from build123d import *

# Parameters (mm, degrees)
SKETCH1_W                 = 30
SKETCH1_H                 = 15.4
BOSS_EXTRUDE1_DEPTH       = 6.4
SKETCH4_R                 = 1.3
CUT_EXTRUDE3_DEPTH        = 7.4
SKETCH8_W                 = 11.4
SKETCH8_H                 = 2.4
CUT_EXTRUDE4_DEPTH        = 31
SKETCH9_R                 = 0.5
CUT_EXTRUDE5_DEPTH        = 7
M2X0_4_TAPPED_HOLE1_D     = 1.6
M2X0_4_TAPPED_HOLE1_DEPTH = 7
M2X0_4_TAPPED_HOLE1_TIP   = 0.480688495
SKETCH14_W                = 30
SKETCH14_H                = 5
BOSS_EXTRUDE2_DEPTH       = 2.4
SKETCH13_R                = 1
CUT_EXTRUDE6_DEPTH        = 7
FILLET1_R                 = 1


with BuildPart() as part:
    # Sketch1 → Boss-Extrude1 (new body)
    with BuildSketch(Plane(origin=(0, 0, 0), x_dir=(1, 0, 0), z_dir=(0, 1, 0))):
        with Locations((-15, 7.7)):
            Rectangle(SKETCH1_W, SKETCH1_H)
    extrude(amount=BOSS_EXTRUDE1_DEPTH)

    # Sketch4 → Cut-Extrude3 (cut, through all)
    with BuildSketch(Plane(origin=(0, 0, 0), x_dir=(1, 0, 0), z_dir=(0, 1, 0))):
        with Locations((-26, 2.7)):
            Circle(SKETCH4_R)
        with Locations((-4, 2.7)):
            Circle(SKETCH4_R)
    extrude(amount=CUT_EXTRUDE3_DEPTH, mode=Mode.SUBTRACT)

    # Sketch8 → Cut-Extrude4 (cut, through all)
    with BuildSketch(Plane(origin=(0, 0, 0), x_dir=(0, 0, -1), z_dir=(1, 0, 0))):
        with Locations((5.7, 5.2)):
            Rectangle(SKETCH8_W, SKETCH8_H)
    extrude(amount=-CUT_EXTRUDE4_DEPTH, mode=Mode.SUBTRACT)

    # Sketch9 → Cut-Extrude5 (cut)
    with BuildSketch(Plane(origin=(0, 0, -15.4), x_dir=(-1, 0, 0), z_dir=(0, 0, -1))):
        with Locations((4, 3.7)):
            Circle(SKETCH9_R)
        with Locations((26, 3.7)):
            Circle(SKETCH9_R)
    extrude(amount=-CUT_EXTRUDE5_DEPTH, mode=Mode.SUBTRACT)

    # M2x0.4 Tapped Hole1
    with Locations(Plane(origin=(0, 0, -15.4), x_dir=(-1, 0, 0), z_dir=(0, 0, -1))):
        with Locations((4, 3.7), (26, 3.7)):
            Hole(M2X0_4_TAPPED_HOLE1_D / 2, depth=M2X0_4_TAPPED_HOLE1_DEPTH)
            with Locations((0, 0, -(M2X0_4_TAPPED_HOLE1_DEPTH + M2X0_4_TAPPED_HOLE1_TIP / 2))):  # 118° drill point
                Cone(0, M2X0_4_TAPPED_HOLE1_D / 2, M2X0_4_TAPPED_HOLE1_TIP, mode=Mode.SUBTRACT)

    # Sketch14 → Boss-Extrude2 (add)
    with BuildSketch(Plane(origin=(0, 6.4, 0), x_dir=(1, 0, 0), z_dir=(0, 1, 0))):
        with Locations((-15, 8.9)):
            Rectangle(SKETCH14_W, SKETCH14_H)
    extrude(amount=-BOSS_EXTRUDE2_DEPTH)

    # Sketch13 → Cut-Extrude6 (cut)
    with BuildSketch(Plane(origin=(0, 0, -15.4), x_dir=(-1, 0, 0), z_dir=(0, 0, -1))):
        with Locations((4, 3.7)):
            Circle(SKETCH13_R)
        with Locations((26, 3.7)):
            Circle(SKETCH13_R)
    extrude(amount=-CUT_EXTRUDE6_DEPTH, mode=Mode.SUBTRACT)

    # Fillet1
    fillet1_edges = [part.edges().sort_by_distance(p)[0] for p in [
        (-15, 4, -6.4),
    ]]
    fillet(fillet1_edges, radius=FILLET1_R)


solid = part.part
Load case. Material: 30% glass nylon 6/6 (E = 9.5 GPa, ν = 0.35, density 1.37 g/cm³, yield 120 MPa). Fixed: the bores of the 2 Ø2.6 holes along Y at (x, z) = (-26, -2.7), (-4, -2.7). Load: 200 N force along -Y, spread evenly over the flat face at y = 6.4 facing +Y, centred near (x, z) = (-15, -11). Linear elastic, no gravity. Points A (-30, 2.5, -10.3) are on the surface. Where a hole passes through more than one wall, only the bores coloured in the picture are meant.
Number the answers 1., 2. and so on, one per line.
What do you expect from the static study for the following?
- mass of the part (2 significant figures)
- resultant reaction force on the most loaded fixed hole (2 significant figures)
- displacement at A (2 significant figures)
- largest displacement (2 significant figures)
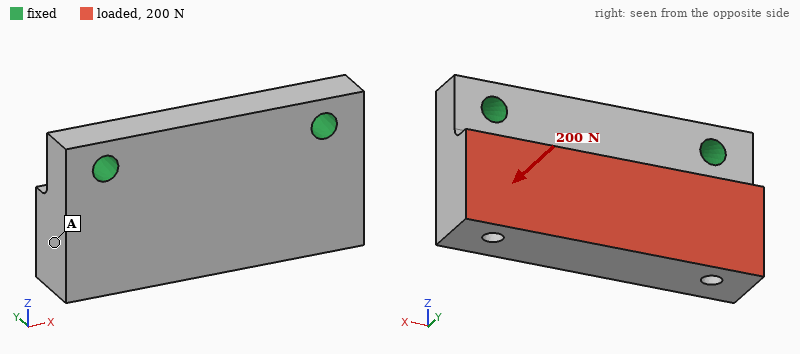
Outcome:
1. 3.3 g
2. 100 N
3. 31 µm
4. 77 µm
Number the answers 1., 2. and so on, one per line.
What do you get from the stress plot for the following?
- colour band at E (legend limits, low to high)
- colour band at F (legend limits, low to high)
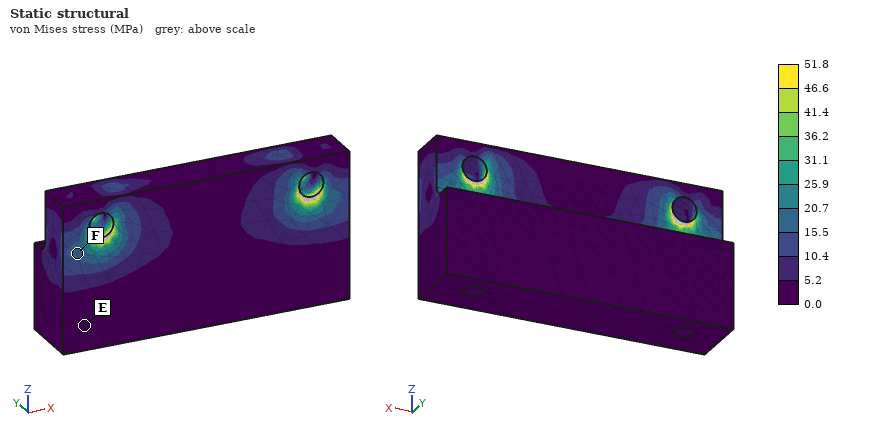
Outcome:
1. 0.0 to 5.2 MPa
2. 15.5 to 20.7 MPa
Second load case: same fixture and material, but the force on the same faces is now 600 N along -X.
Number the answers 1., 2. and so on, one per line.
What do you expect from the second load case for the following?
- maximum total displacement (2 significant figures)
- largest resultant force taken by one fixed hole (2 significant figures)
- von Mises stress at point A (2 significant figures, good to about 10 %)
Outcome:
1. 41 µm
2. 380 N
3. 3.5 MPa
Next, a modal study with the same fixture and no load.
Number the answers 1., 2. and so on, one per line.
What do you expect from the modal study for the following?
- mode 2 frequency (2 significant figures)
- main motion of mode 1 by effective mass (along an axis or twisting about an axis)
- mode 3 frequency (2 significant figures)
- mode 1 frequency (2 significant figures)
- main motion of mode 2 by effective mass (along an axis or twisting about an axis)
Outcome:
1. 13 kHz
2. along Y
3. 20 kHz
4. 6500 Hz
5. twisting about Z
